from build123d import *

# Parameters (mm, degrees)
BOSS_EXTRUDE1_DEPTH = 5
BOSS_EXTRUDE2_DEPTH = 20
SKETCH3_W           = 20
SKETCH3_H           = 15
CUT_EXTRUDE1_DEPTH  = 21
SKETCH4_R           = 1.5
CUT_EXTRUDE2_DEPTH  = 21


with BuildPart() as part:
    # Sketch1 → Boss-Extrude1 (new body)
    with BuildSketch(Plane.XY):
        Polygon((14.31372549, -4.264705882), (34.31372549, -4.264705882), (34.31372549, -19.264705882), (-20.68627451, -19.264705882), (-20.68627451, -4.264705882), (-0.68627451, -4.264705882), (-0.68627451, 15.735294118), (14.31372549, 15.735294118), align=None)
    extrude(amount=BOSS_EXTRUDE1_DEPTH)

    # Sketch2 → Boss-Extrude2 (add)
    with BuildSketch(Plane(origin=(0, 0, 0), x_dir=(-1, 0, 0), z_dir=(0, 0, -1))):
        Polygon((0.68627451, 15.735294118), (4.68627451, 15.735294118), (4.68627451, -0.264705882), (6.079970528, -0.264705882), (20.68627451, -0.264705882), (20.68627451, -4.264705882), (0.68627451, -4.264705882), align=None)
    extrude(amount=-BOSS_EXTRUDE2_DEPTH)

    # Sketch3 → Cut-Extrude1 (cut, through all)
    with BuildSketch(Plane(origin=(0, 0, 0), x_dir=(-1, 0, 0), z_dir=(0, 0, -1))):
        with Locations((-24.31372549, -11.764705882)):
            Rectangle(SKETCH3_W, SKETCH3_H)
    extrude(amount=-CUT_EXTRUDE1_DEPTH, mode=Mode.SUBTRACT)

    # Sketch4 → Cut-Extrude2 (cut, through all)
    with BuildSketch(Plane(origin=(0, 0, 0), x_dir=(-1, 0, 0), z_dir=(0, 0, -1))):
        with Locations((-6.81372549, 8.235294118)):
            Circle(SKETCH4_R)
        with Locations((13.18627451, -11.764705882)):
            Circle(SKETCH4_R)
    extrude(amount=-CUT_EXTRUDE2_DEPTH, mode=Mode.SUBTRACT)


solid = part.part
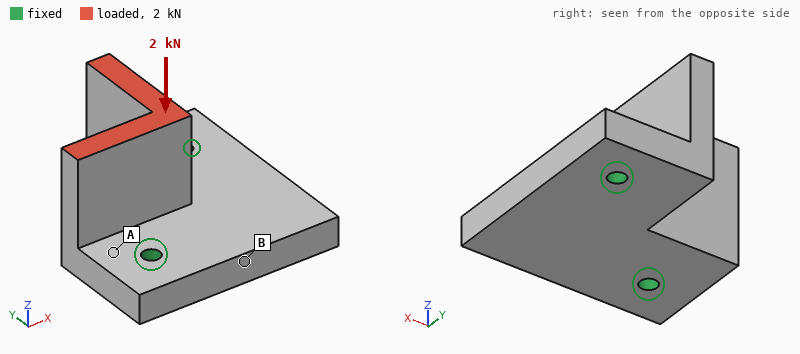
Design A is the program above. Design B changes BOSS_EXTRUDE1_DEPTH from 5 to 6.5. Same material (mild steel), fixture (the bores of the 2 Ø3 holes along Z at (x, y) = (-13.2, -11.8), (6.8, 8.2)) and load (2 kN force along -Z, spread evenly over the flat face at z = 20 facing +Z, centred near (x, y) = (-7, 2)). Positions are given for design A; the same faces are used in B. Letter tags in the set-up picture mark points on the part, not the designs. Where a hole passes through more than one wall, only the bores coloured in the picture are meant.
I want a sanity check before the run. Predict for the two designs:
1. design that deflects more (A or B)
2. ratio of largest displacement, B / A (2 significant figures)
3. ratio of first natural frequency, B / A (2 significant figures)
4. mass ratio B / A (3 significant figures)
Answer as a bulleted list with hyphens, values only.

- A
- 0.58
- 1.3
- 1.18
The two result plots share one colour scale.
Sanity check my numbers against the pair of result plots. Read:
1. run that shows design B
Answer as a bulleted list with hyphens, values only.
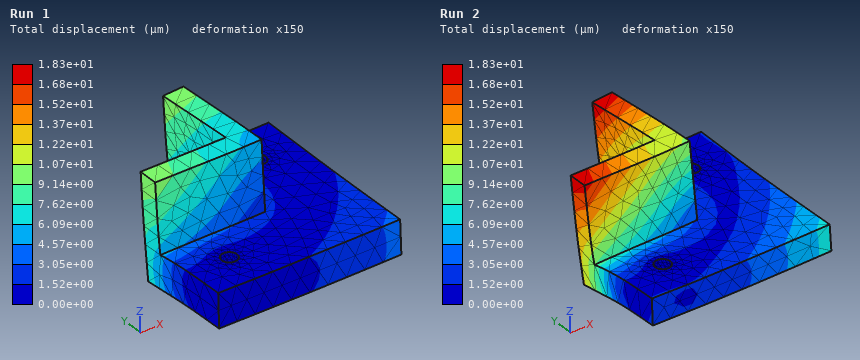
- Run 1
